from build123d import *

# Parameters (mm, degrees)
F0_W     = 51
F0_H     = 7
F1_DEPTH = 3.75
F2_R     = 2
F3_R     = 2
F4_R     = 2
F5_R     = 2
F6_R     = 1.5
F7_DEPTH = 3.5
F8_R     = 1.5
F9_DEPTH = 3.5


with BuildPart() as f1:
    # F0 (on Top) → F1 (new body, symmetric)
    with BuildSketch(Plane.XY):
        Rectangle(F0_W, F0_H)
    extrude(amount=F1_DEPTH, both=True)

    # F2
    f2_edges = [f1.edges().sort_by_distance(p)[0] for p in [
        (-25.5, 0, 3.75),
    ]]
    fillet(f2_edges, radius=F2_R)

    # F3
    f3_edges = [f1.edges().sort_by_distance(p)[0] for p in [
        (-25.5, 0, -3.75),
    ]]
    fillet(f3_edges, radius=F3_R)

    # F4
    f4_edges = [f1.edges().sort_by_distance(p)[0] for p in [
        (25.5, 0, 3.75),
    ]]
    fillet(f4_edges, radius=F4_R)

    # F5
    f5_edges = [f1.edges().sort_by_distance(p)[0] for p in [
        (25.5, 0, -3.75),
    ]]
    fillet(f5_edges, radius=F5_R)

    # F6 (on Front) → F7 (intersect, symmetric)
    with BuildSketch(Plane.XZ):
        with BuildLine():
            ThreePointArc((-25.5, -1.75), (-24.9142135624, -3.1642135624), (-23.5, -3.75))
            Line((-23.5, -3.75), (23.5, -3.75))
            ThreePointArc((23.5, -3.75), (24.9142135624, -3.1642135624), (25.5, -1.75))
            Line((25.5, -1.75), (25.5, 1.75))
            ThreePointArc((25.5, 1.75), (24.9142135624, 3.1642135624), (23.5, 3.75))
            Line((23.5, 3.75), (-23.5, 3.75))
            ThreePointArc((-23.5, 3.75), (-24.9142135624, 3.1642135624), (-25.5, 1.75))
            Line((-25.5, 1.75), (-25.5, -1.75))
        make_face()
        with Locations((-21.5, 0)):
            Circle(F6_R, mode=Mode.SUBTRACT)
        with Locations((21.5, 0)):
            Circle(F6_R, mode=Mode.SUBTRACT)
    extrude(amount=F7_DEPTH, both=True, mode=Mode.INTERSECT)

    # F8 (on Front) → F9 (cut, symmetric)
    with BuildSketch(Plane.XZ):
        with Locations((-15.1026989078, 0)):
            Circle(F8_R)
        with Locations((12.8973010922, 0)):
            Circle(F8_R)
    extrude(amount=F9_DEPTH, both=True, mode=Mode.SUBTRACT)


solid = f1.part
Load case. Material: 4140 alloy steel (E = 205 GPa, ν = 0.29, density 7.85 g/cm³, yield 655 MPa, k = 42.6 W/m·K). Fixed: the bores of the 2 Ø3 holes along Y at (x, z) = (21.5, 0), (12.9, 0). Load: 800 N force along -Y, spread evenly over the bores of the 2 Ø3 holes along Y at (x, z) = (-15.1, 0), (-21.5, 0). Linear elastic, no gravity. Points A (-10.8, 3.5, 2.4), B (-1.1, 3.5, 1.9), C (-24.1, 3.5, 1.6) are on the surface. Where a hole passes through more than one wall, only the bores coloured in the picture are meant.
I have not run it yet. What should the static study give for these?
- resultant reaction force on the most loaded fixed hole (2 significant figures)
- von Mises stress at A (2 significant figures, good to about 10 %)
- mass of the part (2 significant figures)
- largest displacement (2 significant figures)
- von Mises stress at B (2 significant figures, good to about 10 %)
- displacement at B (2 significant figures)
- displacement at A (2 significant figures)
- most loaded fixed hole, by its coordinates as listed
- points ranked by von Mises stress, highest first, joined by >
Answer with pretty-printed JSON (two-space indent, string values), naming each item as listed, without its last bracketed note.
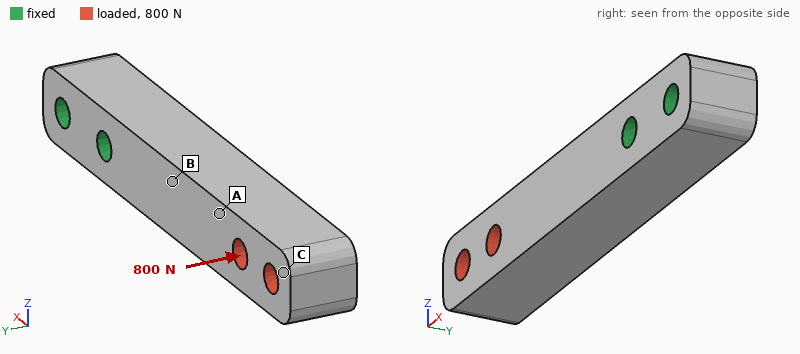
{
  "resultant reaction force on the most loaded fixed hole": "1.1 kN",
  "von Mises stress at A": "100 MPa",
  "mass of the part": "19 g",
  "largest displacement": "0.25 mm",
  "von Mises stress at B": "220 MPa",
  "displacement at B": "0.052 mm",
  "displacement at A": "0.12 mm",
  "most loaded fixed hole, by its coordinates as listed": "(12.9, 0)",
  "points ranked by von Mises stress, highest first, joined by >": "B > A > C"
}
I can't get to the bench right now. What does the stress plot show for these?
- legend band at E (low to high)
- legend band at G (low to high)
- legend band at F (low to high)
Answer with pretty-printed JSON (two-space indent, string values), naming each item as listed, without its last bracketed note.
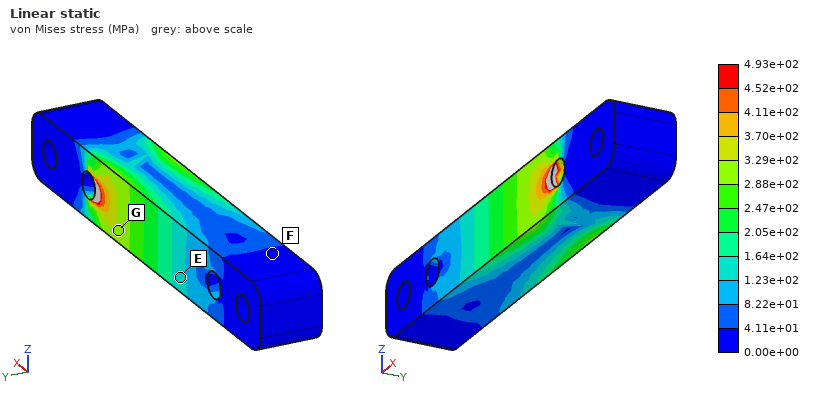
{
  "legend band at E": "1.23e+02 to 1.64e+02 MPa",
  "legend band at G": "2.88e+02 to 3.29e+02 MPa",
  "legend band at F": "0.00e+00 to 4.11e+01 MPa"
}
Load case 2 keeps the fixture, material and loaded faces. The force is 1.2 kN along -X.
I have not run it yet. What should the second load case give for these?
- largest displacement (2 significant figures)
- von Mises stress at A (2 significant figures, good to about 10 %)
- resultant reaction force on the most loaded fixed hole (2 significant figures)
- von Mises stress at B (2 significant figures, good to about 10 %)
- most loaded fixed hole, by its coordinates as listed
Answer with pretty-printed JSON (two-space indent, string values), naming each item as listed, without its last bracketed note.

{
  "largest displacement": "3.9 µm",
  "von Mises stress at A": "24 MPa",
  "resultant reaction force on the most loaded fixed hole": "1.1 kN",
  "von Mises stress at B": "23 MPa",
  "most loaded fixed hole, by its coordinates as listed": "(12.9, 0)"
}
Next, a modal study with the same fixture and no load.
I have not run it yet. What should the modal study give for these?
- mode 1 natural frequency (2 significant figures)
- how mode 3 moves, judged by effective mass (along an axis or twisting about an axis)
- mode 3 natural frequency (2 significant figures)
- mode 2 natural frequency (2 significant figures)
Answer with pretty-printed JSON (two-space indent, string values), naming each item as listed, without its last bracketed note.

{
  "mode 1 natural frequency": "4100 Hz",
  "how mode 3 moves, judged by effective mass": "twisting about X",
  "mode 3 natural frequency": "20 kHz",
  "mode 2 natural frequency": "4200 Hz"
}
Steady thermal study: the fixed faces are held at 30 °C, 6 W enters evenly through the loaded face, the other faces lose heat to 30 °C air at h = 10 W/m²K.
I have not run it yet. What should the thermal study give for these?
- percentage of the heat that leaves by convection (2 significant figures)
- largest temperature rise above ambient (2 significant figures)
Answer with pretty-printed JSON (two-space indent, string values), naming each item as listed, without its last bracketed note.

{
  "percentage of the heat that leaves by convection": "8.5 %",
  "largest temperature rise above ambient": "83 K"
}
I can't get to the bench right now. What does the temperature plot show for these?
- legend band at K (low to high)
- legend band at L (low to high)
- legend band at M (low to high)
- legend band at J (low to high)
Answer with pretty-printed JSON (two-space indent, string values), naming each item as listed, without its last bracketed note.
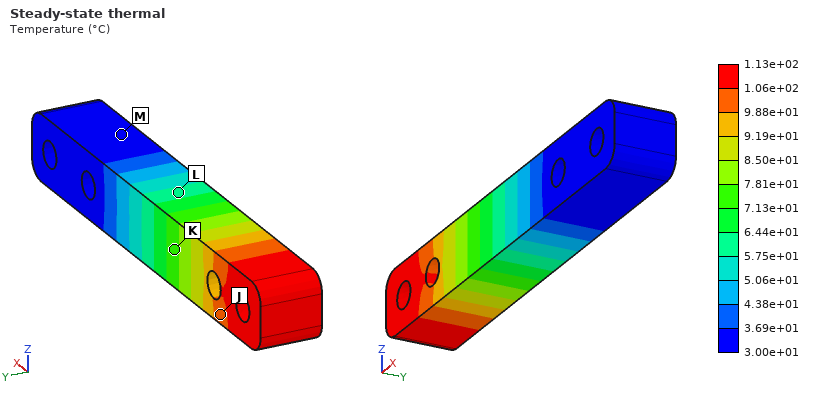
{
  "legend band at K": "7.13e+01 to 7.81e+01 °C",
  "legend band at L": "5.75e+01 to 6.44e+01 °C",
  "legend band at M": "3.00e+01 to 3.69e+01 °C",
  "legend band at J": "9.88e+01 to 1.06e+02 °C"
}
